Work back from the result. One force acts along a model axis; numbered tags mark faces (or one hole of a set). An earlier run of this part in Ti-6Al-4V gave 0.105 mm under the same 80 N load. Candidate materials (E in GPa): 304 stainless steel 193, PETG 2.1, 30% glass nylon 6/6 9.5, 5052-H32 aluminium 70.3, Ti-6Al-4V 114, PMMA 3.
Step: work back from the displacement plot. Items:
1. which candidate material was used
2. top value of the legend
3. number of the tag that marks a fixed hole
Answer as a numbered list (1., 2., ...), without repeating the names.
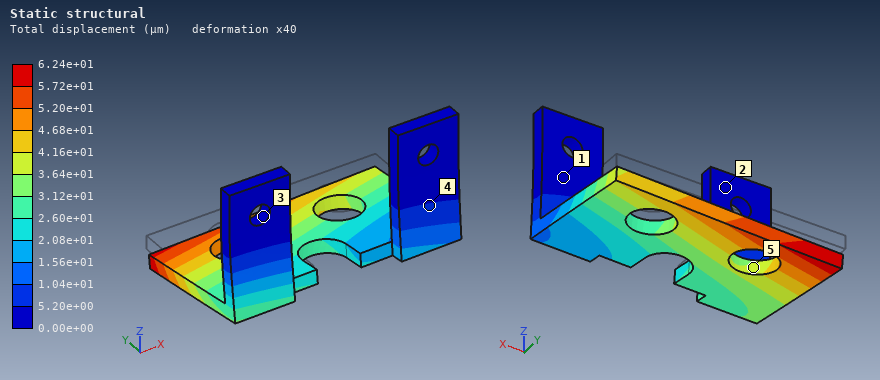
1. 304 stainless steel
2. 6.24e+01 µm
3. 3
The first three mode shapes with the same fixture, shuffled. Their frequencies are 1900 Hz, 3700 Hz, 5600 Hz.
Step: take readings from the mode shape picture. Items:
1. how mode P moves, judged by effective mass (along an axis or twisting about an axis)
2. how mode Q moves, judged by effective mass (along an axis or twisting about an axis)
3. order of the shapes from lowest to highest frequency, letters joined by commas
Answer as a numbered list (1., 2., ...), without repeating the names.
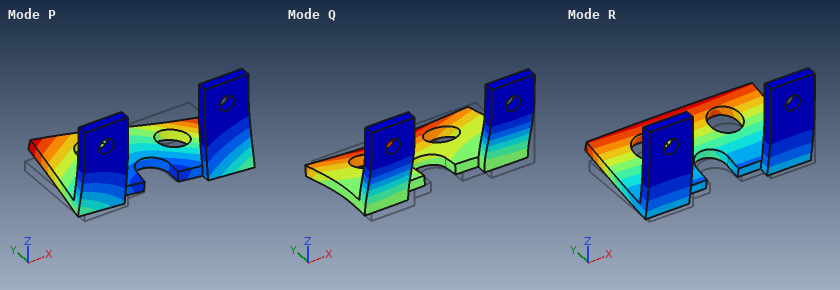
1. along X
2. along Y
3. R, P, Q
